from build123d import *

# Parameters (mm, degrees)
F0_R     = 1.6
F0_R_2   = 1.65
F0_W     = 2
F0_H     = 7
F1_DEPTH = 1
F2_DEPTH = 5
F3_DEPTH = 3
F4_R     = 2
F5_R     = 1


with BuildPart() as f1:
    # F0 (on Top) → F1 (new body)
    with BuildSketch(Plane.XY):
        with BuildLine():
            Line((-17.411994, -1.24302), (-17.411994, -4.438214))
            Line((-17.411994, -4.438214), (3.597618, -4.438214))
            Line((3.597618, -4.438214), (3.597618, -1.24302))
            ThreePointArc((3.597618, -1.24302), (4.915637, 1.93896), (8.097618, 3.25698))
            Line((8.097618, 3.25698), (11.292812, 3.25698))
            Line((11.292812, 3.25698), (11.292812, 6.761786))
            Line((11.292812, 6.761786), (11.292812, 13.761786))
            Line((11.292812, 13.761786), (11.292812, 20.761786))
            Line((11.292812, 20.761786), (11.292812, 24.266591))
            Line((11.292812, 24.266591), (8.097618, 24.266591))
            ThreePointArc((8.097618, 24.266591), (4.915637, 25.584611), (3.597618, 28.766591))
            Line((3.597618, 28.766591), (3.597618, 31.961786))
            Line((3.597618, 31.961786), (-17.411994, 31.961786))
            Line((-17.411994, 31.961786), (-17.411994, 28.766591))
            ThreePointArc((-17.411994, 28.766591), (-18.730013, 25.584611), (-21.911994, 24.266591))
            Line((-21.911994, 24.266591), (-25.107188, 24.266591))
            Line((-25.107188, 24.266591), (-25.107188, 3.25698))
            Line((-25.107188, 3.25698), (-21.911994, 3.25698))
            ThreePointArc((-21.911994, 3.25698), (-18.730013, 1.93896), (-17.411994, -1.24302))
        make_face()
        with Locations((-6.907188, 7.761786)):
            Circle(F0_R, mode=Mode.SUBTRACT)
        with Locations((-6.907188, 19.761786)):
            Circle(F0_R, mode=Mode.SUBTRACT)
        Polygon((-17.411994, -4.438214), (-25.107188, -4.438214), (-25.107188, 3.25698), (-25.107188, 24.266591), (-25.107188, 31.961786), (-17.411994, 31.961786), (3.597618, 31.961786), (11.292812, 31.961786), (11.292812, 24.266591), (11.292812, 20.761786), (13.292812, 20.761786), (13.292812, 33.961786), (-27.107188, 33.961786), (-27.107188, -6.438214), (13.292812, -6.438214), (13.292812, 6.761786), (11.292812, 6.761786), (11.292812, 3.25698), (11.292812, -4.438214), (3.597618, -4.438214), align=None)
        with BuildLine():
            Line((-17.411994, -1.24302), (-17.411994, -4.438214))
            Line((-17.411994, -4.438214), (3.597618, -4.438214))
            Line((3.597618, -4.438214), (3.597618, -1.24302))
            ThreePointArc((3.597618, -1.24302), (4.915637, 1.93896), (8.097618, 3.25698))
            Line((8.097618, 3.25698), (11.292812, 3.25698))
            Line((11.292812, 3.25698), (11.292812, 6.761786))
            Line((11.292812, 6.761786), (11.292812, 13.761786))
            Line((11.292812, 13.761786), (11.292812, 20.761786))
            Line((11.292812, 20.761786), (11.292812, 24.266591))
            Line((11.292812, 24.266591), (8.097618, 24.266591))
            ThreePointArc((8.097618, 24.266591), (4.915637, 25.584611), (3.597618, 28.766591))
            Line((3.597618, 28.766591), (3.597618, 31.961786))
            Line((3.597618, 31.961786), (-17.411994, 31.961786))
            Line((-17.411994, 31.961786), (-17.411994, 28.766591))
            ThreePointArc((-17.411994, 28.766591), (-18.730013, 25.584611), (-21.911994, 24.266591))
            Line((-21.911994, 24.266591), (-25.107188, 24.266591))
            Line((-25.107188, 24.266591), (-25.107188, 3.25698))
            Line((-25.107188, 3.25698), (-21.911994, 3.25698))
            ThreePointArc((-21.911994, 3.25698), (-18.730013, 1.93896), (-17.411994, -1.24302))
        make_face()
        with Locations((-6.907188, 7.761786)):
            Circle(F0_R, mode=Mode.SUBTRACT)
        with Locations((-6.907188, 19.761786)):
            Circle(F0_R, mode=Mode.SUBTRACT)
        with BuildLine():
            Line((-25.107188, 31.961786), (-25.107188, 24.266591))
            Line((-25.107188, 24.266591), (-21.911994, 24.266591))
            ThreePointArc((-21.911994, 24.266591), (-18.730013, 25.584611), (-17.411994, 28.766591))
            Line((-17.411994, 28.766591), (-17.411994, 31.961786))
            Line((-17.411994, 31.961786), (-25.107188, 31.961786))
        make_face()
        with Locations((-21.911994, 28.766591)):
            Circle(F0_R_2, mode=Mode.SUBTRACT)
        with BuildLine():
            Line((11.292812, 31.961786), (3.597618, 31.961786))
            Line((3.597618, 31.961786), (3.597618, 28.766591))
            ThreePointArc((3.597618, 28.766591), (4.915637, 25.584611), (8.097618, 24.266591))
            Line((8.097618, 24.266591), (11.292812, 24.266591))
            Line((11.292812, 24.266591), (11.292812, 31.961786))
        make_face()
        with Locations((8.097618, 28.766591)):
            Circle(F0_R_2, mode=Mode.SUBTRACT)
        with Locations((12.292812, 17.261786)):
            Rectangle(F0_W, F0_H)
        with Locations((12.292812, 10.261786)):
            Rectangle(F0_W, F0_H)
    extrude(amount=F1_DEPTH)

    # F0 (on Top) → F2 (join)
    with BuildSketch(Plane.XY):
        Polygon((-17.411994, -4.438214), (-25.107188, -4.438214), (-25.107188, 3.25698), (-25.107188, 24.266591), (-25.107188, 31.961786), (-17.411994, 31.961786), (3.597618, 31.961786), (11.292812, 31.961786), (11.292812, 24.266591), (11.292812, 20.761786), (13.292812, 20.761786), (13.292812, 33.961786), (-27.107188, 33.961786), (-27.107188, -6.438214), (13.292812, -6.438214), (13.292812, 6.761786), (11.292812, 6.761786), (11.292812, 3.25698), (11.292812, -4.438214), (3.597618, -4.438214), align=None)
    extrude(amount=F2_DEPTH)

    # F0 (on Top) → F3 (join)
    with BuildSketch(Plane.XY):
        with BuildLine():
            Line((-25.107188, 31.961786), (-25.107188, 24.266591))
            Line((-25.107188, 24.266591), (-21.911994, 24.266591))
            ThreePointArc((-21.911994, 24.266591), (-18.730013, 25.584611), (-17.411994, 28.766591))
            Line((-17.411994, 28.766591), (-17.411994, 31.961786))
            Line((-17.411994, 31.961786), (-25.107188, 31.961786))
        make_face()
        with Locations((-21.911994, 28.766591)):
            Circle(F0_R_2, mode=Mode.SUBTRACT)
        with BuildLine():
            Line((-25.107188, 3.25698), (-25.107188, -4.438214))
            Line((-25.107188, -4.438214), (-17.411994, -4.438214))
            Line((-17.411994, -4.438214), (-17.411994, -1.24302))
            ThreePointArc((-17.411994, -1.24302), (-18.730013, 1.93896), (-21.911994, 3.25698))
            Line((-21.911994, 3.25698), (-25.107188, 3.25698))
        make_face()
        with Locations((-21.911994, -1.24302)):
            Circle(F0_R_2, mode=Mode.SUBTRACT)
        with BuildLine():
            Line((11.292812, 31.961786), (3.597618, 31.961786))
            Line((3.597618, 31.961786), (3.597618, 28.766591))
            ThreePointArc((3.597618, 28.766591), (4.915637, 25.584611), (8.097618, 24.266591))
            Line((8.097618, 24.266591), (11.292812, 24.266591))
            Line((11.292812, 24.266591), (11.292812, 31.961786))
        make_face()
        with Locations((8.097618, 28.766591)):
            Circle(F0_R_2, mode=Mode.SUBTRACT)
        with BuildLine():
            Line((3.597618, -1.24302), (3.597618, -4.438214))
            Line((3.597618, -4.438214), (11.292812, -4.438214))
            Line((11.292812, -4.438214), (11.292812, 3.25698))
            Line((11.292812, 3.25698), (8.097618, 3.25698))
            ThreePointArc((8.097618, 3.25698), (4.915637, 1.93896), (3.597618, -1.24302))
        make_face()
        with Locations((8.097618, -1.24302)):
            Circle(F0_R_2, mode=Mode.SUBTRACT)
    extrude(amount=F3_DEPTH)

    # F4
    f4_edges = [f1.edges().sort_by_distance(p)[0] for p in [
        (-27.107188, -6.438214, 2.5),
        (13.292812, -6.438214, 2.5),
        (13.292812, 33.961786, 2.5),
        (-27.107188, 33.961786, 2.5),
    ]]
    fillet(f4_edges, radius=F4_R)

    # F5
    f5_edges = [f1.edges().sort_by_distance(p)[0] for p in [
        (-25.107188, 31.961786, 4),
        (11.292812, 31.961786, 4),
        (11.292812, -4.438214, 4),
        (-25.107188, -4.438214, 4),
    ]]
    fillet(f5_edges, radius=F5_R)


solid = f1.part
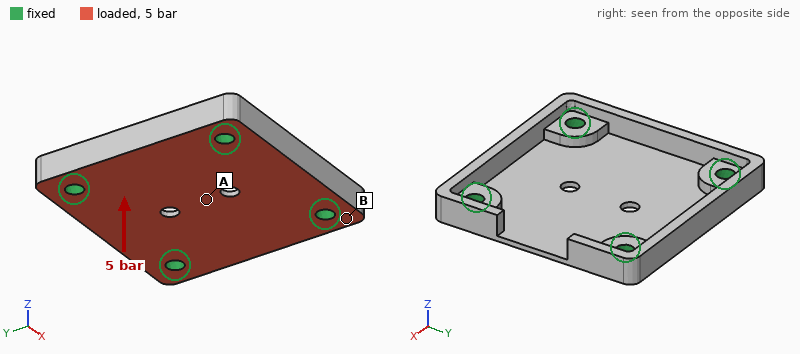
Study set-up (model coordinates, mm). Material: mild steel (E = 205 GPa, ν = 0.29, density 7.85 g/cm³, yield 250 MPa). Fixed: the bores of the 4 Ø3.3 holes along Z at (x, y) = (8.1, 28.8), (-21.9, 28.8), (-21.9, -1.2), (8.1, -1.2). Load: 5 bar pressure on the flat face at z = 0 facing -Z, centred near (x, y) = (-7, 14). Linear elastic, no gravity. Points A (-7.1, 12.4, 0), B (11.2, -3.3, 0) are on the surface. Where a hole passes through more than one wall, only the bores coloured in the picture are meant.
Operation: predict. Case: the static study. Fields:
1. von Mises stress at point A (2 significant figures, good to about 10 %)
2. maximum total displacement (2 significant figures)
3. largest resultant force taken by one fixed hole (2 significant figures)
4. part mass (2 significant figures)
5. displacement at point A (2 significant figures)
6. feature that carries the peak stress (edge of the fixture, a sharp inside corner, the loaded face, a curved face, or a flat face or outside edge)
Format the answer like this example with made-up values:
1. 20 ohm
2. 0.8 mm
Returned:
1. 86 MPa
2. 58 µm
3. 220 N
4. 24 g
5. 57 µm
6. the loaded face
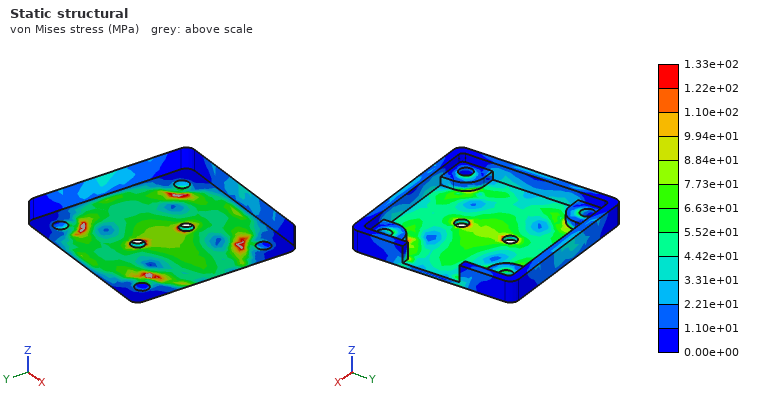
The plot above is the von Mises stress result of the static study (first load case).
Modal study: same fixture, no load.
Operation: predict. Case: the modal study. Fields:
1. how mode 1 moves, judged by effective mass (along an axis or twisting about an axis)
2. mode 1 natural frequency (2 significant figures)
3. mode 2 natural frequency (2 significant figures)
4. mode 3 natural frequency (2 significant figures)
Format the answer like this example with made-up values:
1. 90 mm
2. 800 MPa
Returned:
1. along Z
2. 6800 Hz
3. 13 kHz
4. 14 kHz
